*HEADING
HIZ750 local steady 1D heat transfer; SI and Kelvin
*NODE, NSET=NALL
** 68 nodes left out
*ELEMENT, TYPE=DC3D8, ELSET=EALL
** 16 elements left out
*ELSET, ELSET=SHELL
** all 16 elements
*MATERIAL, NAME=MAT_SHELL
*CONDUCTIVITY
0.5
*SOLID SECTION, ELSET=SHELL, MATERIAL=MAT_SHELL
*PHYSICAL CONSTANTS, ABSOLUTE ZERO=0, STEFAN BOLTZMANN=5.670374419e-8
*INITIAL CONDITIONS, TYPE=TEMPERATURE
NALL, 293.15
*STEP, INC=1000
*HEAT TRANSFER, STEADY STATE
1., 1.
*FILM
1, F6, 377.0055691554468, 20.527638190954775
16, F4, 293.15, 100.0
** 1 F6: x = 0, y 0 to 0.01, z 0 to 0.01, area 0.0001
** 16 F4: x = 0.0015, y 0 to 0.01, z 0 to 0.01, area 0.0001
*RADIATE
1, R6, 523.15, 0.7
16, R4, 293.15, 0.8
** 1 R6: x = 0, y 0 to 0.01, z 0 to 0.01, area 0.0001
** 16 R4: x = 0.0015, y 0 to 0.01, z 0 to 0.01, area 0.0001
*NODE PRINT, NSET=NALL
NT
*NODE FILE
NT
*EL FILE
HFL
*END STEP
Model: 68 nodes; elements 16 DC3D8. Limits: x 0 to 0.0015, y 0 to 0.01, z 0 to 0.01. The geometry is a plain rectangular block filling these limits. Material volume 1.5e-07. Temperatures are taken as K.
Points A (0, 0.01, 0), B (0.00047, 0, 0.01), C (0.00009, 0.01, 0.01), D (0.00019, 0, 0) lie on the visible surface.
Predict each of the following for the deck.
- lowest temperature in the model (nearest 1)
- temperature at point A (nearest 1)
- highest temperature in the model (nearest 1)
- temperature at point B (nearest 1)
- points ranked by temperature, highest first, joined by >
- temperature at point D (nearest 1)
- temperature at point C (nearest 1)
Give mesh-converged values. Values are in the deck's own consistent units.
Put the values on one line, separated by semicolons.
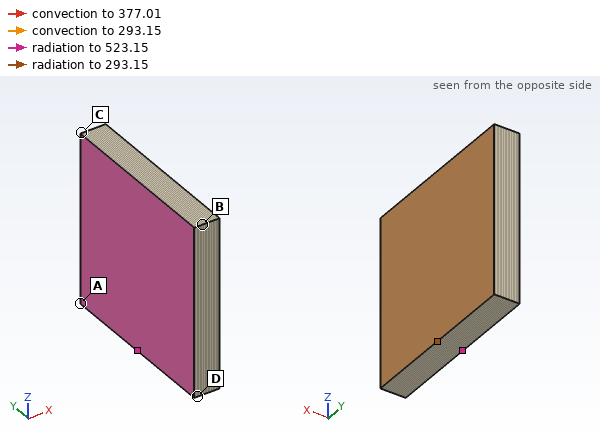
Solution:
325 K; 335 K; 335 K; 332 K; A > C > D > B; 334 K; 334 K
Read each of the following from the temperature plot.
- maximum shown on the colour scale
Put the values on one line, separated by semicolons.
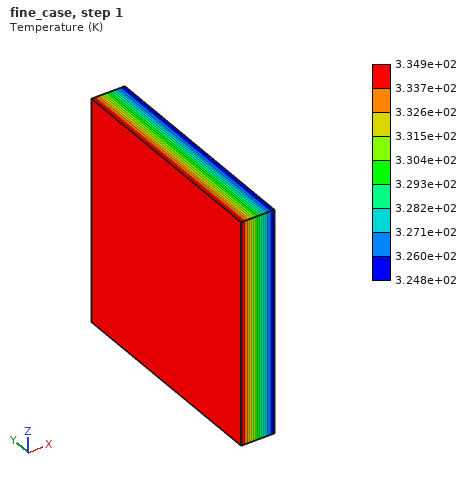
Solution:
3.349e+02 K
